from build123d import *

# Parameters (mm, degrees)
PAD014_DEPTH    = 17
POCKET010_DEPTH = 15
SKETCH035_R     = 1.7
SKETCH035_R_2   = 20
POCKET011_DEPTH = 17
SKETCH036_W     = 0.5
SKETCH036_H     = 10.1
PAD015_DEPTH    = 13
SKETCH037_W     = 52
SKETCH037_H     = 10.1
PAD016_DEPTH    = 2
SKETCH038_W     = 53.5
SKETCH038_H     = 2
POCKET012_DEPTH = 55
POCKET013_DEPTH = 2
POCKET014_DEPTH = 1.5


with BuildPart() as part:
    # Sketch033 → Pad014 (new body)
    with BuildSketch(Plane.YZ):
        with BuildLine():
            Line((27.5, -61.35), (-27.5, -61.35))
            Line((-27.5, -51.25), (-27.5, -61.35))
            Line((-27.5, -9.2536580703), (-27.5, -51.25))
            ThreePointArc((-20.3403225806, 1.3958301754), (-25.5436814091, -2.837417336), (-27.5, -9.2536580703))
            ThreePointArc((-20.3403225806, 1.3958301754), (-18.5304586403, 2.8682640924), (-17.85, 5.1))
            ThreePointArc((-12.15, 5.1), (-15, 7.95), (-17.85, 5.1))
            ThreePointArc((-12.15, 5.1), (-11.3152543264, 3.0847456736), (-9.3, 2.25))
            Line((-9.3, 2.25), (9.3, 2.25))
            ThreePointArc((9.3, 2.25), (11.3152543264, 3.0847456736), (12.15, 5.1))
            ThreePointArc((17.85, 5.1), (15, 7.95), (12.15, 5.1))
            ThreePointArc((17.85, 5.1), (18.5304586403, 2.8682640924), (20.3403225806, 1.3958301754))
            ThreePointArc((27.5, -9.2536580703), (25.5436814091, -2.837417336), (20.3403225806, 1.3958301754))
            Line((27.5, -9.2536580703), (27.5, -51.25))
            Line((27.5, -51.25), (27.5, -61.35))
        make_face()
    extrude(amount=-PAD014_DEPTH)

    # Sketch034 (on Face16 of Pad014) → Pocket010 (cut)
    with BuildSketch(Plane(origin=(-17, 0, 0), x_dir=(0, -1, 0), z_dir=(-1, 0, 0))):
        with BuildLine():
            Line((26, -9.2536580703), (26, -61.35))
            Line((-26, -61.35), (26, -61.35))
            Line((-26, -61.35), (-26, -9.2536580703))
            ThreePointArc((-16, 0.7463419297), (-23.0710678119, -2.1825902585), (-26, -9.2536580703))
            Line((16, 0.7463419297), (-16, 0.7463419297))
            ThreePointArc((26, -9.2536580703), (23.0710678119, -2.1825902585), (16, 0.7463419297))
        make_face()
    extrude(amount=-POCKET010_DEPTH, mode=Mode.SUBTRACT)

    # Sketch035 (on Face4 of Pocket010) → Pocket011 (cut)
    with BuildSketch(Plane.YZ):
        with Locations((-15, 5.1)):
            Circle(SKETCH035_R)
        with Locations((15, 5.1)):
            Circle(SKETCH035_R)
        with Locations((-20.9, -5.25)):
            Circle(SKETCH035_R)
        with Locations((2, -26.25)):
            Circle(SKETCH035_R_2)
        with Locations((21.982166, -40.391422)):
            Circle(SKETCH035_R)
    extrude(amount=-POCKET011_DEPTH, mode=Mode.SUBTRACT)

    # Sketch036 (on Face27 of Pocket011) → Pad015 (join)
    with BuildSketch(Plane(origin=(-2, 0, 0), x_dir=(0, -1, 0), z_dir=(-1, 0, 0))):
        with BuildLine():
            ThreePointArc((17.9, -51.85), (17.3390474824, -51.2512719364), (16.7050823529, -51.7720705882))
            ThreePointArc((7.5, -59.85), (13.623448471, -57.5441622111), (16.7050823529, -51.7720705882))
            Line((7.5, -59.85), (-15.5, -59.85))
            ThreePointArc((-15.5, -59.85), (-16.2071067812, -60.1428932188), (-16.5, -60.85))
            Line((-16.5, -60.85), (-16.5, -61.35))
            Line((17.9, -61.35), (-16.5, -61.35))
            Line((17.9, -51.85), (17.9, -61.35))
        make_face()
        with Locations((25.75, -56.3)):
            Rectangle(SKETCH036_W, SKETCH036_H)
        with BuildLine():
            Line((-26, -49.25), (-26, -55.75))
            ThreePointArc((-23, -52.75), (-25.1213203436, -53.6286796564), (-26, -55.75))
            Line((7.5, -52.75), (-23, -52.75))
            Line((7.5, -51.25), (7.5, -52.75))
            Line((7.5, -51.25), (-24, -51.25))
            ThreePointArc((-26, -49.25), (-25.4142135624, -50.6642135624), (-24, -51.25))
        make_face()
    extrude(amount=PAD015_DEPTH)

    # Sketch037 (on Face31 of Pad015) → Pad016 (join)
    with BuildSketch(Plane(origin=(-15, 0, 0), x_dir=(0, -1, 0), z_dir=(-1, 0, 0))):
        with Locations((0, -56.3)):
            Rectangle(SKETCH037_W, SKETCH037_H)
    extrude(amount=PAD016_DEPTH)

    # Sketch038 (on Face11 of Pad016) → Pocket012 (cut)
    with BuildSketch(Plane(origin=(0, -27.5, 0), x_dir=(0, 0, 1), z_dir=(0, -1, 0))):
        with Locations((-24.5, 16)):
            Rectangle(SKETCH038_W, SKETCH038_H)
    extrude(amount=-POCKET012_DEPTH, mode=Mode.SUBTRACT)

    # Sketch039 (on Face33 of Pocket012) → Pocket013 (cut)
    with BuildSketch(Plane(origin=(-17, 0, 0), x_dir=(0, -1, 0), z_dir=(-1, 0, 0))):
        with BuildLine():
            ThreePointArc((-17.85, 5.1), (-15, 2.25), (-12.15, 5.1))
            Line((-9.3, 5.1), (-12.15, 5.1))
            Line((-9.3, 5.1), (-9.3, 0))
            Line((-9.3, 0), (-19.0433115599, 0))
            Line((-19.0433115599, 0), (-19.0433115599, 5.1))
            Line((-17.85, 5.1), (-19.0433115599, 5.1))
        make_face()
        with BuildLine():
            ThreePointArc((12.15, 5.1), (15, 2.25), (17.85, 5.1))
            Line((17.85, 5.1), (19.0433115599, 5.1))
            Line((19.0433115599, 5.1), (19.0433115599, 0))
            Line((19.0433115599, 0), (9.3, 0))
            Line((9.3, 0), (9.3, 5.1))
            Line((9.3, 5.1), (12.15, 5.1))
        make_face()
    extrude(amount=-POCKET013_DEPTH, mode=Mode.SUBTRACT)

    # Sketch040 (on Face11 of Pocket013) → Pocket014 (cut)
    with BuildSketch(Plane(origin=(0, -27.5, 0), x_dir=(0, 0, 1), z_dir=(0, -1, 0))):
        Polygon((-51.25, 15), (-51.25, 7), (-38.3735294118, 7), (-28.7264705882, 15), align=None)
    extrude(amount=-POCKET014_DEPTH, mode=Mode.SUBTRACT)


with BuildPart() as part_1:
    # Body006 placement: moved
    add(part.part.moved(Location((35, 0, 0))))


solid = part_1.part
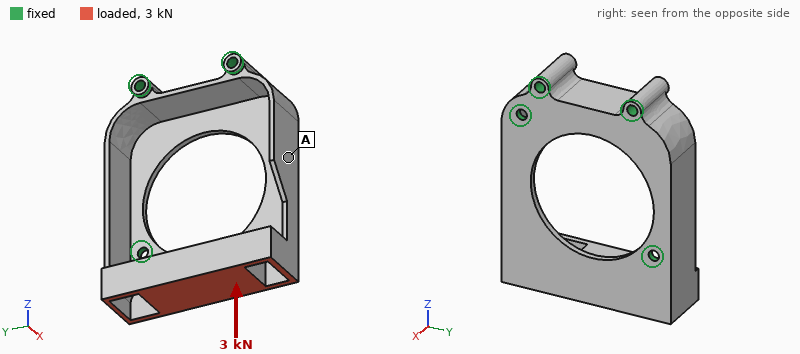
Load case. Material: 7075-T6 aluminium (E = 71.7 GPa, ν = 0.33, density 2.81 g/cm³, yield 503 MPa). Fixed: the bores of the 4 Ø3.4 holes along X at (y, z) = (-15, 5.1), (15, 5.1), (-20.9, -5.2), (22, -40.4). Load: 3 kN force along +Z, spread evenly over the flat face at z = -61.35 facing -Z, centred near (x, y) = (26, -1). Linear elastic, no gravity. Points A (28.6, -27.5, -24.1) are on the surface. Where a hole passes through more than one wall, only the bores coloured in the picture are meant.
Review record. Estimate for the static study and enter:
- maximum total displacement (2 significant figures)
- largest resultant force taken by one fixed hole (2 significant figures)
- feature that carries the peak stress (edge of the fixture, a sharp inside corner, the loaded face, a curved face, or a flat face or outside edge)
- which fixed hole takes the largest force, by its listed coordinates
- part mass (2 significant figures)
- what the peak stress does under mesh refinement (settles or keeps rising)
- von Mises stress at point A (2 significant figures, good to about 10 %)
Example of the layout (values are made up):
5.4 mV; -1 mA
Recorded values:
0.67 mm; 1.6 kN; a sharp inside corner; (-20.9, -5.2); 31 g; keeps rising; 44 MPa
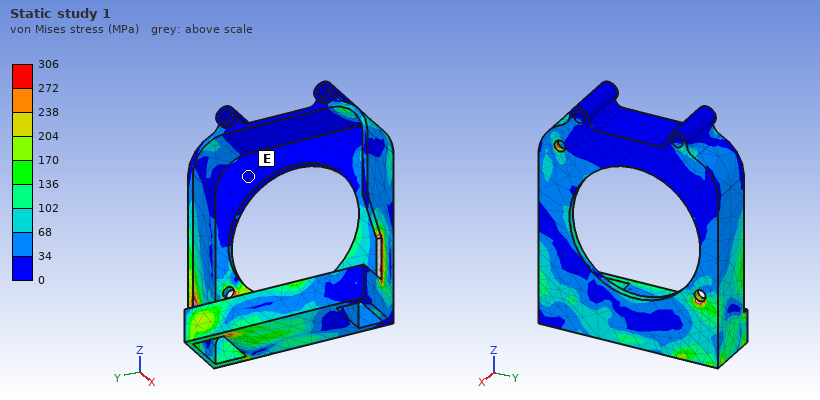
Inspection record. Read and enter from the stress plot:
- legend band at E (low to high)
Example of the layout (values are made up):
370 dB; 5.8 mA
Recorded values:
0 to 34 MPa
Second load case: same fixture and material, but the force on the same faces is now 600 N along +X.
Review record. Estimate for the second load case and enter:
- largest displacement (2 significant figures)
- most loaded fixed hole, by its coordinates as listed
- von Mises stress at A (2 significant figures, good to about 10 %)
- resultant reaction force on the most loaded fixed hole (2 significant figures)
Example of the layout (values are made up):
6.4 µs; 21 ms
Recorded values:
0.97 mm; (-20.9, -5.2); 78 MPa; 820 N
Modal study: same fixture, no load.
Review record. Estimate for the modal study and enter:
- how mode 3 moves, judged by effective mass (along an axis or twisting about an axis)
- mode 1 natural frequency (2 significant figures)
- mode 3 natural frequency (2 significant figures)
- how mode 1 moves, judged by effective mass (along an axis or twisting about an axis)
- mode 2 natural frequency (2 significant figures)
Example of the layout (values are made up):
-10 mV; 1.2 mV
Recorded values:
along Y; 1300 Hz; 6100 Hz; along X; 4200 Hz
